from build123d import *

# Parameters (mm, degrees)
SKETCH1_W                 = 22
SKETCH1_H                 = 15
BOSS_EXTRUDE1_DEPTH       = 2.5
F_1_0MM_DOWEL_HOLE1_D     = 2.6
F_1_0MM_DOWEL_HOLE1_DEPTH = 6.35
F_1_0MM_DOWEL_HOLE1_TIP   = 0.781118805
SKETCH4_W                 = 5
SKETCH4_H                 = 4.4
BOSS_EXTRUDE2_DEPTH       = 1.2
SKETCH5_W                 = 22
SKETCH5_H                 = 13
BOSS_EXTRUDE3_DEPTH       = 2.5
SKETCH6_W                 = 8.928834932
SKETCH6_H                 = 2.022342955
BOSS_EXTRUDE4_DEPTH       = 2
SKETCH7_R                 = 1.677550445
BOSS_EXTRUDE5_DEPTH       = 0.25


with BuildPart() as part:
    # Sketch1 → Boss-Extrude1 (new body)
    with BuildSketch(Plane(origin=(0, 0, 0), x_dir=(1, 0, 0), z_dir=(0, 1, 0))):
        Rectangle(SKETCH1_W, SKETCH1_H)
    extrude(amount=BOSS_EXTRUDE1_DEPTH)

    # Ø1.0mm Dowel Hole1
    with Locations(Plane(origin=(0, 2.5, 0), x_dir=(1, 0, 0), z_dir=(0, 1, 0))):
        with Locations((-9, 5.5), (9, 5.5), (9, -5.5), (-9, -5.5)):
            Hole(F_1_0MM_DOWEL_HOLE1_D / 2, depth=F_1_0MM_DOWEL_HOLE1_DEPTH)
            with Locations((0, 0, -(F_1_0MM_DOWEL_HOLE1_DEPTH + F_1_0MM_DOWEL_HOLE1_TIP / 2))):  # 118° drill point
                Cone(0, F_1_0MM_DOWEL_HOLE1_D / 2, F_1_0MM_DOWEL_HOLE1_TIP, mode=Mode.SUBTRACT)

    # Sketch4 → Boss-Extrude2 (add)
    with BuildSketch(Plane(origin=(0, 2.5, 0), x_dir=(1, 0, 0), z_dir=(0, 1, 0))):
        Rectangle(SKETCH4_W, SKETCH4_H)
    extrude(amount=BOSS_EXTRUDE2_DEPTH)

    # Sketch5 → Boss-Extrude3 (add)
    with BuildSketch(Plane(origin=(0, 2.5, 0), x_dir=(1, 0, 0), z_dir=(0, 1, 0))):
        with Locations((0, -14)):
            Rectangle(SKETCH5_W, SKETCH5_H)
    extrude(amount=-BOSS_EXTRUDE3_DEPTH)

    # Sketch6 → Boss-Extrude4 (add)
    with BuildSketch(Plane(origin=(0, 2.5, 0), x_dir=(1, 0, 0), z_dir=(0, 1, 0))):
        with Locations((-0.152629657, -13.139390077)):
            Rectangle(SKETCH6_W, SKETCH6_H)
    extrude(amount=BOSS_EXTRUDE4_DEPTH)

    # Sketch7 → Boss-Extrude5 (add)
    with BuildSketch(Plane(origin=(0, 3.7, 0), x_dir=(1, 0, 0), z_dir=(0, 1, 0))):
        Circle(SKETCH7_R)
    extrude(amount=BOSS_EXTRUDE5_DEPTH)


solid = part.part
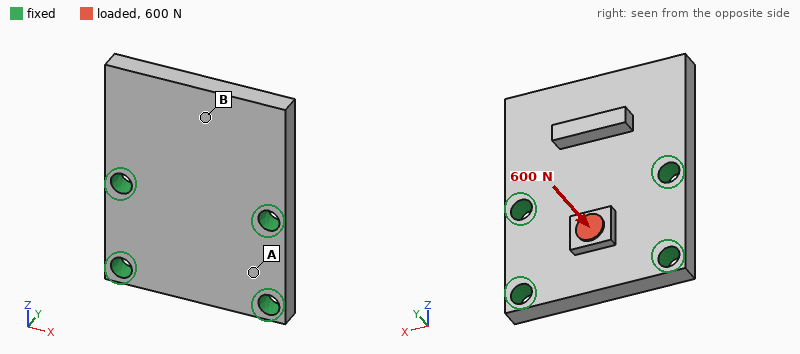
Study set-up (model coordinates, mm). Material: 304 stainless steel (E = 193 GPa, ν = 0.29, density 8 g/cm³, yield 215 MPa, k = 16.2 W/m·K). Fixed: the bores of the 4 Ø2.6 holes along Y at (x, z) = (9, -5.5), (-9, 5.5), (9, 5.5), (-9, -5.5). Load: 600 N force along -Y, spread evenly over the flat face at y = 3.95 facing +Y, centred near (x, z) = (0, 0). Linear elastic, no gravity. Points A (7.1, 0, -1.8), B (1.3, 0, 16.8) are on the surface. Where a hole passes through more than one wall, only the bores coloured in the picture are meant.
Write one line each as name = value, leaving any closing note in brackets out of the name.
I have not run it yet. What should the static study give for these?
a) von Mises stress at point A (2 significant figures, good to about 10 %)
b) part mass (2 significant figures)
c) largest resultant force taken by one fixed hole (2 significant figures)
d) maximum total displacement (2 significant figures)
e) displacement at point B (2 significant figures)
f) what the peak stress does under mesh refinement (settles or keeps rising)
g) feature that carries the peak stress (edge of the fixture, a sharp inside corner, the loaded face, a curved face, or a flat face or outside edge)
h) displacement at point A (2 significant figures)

von Mises stress at point A = 26 MPa
part mass = 12 g
largest resultant force taken by one fixed hole = 150 N
maximum total displacement = 5.5 µm
displacement at point B = 1.1 µm
what the peak stress does under mesh refinement = keeps rising
feature that carries the peak stress = edge of the fixture
displacement at point A = 1.4 µm
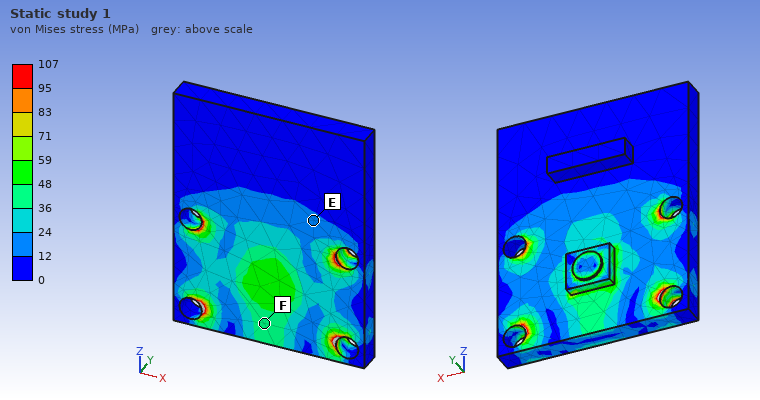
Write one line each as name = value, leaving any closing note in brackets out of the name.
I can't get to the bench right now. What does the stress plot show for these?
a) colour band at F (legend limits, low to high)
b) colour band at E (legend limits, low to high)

colour band at F = 36 to 48 MPa
colour band at E = 12 to 24 MPa
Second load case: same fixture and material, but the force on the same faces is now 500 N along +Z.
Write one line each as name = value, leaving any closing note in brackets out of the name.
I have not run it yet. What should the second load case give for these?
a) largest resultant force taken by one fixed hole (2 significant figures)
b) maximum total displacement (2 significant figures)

largest resultant force taken by one fixed hole = 170 N
maximum total displacement = 3.3 µm
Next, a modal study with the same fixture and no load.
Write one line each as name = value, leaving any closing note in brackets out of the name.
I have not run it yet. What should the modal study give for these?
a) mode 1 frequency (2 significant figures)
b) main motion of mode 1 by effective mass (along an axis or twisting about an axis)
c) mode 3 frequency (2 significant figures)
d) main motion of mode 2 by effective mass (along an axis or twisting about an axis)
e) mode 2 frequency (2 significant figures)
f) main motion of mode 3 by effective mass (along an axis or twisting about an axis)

mode 1 frequency = 8300 Hz
main motion of mode 1 by effective mass = along Y
mode 3 frequency = 34 kHz
main motion of mode 2 by effective mass = twisting about Z
mode 2 frequency = 17 kHz
main motion of mode 3 by effective mass = along Y
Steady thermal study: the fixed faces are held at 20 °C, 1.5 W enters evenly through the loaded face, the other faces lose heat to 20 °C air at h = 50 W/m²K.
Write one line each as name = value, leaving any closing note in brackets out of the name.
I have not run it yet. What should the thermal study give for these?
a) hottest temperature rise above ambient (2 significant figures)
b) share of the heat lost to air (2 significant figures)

hottest temperature rise above ambient = 26 K
share of the heat lost to air = 14 %
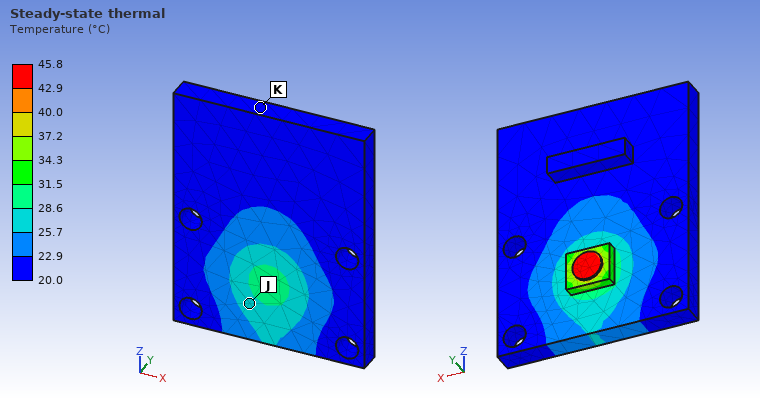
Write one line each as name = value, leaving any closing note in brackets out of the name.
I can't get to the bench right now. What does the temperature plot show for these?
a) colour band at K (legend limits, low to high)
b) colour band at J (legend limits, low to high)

colour band at K = 20.0 to 22.9 °C
colour band at J = 25.7 to 28.6 °C
